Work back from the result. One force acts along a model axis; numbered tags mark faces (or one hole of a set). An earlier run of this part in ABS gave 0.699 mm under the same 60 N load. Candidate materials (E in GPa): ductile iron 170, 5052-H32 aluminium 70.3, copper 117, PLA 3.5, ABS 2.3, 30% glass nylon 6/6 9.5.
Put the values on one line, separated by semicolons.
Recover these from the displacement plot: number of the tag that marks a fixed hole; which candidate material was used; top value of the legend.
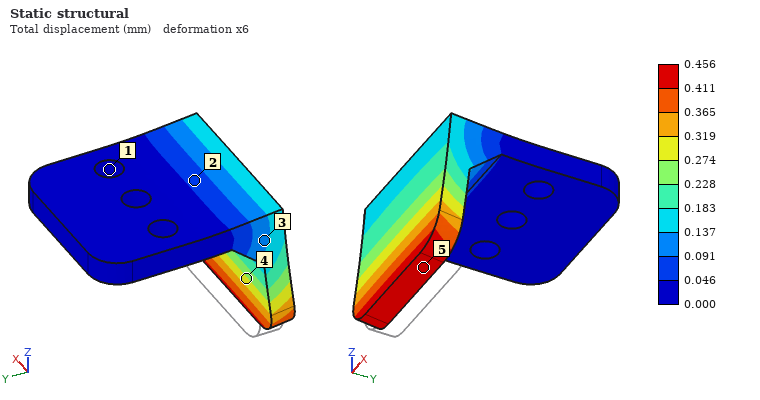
1; PLA; 0.456 mm
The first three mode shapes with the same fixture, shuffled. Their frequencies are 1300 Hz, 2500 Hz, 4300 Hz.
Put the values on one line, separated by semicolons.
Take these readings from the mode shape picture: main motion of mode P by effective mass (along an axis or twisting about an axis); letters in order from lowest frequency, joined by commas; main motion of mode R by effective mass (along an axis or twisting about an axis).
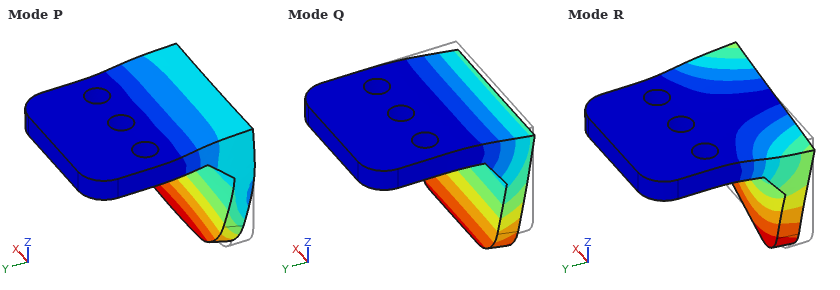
along Z; Q, R, P; along X
